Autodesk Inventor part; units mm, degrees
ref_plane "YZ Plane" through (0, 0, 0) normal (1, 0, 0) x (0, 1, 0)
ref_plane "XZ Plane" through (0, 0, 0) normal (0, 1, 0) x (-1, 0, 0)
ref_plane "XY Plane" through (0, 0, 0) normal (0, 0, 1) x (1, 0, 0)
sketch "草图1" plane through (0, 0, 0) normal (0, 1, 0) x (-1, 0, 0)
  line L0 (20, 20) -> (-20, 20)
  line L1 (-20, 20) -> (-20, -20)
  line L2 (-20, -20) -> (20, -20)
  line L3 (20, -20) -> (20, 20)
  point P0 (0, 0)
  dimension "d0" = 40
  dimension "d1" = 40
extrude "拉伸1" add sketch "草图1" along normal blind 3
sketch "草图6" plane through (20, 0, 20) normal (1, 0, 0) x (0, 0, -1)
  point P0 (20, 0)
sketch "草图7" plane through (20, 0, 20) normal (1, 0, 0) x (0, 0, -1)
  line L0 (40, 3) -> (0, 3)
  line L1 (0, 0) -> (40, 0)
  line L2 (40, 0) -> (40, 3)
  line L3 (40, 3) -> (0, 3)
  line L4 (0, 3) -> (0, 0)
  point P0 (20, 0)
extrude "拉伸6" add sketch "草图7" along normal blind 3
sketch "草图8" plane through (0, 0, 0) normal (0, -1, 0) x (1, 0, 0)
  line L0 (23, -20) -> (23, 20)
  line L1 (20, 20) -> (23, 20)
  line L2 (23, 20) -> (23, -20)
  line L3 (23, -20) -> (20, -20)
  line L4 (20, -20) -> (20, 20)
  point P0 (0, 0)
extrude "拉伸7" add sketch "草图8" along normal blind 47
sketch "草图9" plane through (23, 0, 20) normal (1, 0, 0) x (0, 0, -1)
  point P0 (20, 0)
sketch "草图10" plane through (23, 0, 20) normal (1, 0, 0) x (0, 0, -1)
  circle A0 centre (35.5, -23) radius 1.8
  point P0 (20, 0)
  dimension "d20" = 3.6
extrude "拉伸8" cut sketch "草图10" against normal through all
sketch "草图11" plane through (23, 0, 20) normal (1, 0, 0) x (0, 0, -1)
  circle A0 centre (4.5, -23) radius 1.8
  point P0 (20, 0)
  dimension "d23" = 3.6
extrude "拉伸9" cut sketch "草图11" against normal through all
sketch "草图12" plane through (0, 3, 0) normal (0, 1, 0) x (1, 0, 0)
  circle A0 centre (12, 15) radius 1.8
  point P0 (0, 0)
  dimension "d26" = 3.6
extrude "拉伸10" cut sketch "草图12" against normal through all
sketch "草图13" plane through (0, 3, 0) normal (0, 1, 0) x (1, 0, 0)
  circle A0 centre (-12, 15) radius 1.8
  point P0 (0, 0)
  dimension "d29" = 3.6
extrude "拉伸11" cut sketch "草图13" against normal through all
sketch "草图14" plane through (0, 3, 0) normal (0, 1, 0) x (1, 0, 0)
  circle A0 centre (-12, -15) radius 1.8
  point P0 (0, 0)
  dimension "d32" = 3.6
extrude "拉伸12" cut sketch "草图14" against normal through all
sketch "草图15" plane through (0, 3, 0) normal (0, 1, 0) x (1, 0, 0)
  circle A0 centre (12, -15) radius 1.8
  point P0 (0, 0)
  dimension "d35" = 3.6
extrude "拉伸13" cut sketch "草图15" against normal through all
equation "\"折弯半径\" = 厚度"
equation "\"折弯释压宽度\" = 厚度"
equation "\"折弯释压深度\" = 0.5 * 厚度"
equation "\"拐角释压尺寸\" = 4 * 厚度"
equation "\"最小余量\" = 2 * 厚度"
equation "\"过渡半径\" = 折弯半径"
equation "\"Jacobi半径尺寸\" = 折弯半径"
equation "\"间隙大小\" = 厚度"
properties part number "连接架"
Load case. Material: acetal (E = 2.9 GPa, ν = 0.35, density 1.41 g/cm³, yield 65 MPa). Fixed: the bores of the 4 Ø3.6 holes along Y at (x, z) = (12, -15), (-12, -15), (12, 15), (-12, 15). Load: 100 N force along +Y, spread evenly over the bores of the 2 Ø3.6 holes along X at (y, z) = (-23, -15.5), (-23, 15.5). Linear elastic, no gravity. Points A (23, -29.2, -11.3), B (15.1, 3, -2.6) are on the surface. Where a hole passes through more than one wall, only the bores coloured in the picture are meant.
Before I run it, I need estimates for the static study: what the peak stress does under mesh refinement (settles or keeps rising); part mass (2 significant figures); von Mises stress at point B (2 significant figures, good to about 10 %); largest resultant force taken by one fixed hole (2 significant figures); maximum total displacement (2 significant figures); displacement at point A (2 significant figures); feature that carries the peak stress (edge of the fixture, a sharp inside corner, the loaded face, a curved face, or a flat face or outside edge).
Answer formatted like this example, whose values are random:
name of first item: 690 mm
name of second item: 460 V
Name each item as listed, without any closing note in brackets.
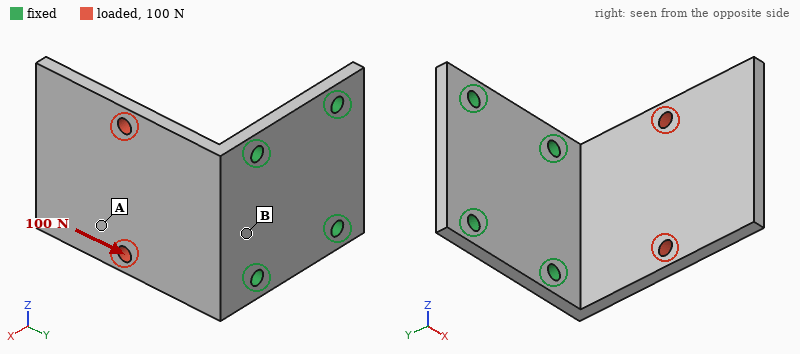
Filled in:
what the peak stress does under mesh refinement: keeps rising
part mass: 15 g
von Mises stress at point B: 4.5 MPa
largest resultant force taken by one fixed hole: 54 N
maximum total displacement: 0.84 mm
displacement at point A: 0.55 mm
feature that carries the peak stress: edge of the fixture
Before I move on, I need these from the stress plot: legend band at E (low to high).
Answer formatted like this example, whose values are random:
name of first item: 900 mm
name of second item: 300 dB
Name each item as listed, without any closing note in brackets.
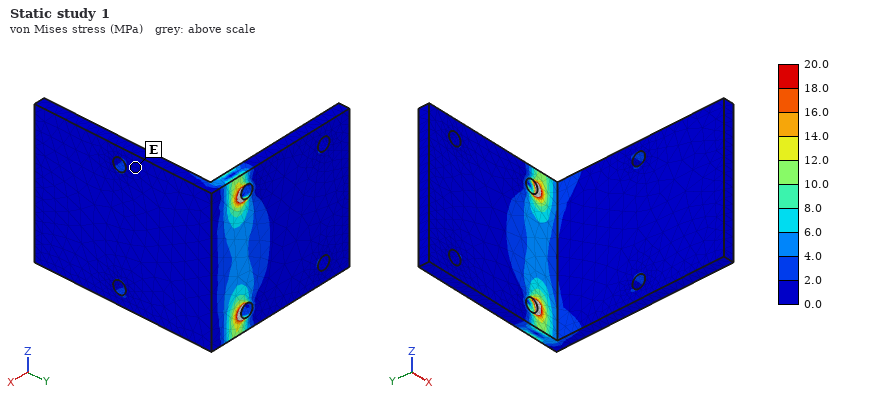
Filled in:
legend band at E: 0.0 to 2.0 MPa
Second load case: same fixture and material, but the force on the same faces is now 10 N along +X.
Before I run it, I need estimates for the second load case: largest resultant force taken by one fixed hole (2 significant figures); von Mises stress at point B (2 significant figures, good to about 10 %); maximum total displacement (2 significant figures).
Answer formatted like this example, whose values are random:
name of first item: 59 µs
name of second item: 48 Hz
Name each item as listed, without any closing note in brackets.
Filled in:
largest resultant force taken by one fixed hole: 3.9 N
von Mises stress at point B: 2.6 MPa
maximum total displacement: 0.79 mm
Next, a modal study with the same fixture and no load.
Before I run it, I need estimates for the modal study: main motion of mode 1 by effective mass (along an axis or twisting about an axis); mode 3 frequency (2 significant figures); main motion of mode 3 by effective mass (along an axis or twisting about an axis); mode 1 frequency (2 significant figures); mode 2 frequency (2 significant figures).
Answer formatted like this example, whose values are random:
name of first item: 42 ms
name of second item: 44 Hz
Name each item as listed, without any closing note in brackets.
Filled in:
main motion of mode 1 by effective mass: along X
mode 3 frequency: 1000 Hz
main motion of mode 3 by effective mass: along Z
mode 1 frequency: 230 Hz
mode 2 frequency: 710 Hz
